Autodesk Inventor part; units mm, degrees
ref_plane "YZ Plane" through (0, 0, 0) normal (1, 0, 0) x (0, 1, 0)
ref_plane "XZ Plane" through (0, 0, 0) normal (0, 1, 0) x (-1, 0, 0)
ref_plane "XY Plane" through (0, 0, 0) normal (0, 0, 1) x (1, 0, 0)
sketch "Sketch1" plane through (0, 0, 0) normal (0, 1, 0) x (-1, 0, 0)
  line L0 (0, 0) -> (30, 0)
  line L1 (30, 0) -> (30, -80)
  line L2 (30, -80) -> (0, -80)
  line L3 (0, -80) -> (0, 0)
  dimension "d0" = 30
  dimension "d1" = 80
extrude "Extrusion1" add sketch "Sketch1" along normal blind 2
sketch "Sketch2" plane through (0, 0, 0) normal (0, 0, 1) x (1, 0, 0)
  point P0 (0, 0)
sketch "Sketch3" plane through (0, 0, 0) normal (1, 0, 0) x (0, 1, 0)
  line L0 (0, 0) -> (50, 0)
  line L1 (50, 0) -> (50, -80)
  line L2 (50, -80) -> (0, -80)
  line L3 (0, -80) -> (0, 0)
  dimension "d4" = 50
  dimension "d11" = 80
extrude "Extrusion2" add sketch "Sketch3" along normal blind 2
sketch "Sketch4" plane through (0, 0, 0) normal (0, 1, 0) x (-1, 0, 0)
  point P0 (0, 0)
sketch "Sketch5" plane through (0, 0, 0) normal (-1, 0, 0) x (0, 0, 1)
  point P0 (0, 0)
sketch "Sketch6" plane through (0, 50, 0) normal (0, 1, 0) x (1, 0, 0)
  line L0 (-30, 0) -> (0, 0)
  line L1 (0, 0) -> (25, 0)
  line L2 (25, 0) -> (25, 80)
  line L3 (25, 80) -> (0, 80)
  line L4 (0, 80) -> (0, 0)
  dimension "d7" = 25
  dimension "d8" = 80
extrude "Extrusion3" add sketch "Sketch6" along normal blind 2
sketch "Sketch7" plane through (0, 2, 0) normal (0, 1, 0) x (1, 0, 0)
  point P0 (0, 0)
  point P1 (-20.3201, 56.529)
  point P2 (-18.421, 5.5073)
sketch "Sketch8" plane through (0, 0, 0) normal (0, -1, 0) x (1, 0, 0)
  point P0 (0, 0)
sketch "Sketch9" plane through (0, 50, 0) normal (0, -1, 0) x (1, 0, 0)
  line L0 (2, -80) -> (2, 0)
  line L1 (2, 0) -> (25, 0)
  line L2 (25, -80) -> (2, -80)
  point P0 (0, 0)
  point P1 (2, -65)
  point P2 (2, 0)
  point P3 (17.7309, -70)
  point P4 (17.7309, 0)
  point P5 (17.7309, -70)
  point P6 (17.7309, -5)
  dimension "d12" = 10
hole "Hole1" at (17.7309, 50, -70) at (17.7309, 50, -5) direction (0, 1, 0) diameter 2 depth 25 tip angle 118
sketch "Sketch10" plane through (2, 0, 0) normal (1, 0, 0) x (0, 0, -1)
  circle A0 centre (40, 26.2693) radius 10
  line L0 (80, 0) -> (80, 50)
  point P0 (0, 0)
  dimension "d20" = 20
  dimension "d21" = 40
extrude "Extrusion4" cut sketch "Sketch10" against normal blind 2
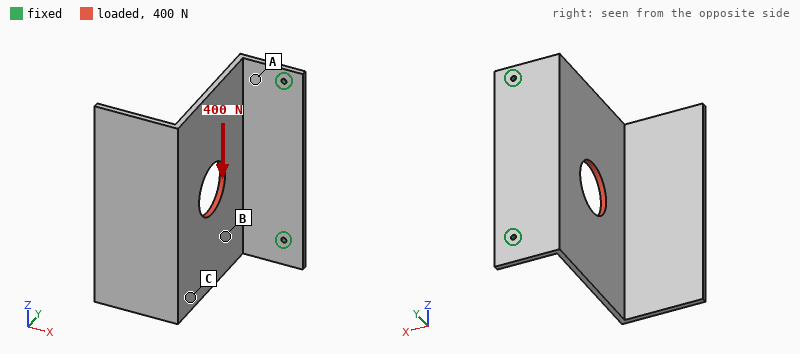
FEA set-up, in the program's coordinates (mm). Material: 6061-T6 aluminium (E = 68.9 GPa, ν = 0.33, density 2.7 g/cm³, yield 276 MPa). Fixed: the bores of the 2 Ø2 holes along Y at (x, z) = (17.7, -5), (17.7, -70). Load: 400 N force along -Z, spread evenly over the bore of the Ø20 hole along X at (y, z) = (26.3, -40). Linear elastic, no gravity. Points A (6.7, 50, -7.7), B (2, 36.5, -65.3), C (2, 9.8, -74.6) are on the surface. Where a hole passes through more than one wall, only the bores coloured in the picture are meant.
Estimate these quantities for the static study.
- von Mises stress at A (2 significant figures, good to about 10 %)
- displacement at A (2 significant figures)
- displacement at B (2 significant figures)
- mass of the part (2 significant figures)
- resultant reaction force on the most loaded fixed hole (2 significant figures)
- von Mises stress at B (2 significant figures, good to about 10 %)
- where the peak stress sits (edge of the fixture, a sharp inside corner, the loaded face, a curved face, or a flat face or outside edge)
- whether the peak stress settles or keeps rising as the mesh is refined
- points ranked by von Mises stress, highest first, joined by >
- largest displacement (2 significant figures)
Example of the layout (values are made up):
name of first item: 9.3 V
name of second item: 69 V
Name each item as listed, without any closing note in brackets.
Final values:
von Mises stress at A: 52 MPa
displacement at A: 0.10 mm
displacement at B: 0.17 mm
mass of the part: 44 g
resultant reaction force on the most loaded fixed hole: 270 N
von Mises stress at B: 24 MPa
where the peak stress sits: edge of the fixture
whether the peak stress settles or keeps rising as the mesh is refined: keeps rising
points ranked by von Mises stress, highest first, joined by >: A > B > C
largest displacement: 0.45 mm
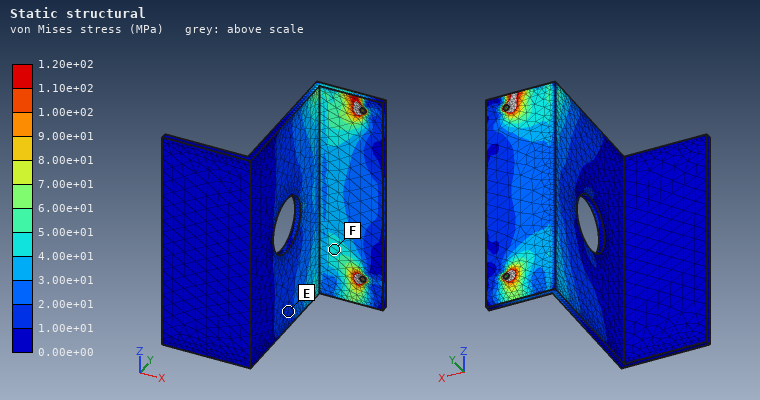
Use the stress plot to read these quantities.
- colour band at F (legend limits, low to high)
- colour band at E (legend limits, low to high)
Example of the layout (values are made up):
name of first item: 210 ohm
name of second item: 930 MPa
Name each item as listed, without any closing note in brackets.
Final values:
colour band at F: 4.00e+01 to 5.00e+01 MPa
colour band at E: 1.00e+01 to 2.00e+01 MPa
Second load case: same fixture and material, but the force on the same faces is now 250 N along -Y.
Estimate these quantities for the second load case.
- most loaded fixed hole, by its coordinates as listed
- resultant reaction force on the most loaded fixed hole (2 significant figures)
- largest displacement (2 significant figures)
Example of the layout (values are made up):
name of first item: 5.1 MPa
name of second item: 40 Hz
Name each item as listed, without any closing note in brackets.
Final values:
most loaded fixed hole, by its coordinates as listed: (17.7, -70)
resultant reaction force on the most loaded fixed hole: 130 N
largest displacement: 1.2 mm
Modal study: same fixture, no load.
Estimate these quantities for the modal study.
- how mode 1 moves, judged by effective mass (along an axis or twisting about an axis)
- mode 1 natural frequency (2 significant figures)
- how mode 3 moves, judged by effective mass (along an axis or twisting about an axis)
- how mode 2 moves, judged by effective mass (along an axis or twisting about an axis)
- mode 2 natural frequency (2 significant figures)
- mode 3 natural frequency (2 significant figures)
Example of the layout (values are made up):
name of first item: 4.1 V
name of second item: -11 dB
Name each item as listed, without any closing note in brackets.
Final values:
how mode 1 moves, judged by effective mass: along X
mode 1 natural frequency: 190 Hz
how mode 3 moves, judged by effective mass: along Z
how mode 2 moves, judged by effective mass: twisting about Y
mode 2 natural frequency: 540 Hz
mode 3 natural frequency: 880 Hz
